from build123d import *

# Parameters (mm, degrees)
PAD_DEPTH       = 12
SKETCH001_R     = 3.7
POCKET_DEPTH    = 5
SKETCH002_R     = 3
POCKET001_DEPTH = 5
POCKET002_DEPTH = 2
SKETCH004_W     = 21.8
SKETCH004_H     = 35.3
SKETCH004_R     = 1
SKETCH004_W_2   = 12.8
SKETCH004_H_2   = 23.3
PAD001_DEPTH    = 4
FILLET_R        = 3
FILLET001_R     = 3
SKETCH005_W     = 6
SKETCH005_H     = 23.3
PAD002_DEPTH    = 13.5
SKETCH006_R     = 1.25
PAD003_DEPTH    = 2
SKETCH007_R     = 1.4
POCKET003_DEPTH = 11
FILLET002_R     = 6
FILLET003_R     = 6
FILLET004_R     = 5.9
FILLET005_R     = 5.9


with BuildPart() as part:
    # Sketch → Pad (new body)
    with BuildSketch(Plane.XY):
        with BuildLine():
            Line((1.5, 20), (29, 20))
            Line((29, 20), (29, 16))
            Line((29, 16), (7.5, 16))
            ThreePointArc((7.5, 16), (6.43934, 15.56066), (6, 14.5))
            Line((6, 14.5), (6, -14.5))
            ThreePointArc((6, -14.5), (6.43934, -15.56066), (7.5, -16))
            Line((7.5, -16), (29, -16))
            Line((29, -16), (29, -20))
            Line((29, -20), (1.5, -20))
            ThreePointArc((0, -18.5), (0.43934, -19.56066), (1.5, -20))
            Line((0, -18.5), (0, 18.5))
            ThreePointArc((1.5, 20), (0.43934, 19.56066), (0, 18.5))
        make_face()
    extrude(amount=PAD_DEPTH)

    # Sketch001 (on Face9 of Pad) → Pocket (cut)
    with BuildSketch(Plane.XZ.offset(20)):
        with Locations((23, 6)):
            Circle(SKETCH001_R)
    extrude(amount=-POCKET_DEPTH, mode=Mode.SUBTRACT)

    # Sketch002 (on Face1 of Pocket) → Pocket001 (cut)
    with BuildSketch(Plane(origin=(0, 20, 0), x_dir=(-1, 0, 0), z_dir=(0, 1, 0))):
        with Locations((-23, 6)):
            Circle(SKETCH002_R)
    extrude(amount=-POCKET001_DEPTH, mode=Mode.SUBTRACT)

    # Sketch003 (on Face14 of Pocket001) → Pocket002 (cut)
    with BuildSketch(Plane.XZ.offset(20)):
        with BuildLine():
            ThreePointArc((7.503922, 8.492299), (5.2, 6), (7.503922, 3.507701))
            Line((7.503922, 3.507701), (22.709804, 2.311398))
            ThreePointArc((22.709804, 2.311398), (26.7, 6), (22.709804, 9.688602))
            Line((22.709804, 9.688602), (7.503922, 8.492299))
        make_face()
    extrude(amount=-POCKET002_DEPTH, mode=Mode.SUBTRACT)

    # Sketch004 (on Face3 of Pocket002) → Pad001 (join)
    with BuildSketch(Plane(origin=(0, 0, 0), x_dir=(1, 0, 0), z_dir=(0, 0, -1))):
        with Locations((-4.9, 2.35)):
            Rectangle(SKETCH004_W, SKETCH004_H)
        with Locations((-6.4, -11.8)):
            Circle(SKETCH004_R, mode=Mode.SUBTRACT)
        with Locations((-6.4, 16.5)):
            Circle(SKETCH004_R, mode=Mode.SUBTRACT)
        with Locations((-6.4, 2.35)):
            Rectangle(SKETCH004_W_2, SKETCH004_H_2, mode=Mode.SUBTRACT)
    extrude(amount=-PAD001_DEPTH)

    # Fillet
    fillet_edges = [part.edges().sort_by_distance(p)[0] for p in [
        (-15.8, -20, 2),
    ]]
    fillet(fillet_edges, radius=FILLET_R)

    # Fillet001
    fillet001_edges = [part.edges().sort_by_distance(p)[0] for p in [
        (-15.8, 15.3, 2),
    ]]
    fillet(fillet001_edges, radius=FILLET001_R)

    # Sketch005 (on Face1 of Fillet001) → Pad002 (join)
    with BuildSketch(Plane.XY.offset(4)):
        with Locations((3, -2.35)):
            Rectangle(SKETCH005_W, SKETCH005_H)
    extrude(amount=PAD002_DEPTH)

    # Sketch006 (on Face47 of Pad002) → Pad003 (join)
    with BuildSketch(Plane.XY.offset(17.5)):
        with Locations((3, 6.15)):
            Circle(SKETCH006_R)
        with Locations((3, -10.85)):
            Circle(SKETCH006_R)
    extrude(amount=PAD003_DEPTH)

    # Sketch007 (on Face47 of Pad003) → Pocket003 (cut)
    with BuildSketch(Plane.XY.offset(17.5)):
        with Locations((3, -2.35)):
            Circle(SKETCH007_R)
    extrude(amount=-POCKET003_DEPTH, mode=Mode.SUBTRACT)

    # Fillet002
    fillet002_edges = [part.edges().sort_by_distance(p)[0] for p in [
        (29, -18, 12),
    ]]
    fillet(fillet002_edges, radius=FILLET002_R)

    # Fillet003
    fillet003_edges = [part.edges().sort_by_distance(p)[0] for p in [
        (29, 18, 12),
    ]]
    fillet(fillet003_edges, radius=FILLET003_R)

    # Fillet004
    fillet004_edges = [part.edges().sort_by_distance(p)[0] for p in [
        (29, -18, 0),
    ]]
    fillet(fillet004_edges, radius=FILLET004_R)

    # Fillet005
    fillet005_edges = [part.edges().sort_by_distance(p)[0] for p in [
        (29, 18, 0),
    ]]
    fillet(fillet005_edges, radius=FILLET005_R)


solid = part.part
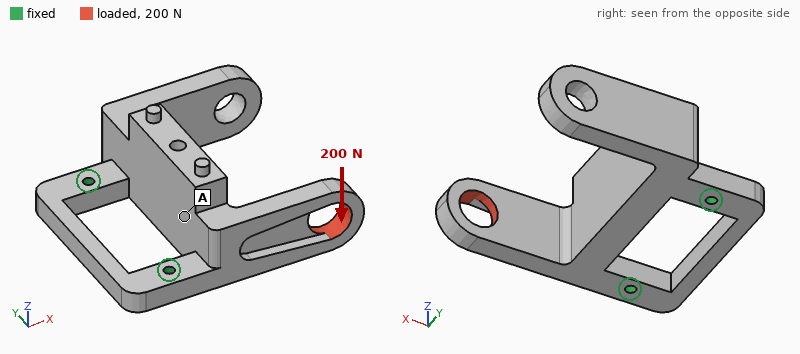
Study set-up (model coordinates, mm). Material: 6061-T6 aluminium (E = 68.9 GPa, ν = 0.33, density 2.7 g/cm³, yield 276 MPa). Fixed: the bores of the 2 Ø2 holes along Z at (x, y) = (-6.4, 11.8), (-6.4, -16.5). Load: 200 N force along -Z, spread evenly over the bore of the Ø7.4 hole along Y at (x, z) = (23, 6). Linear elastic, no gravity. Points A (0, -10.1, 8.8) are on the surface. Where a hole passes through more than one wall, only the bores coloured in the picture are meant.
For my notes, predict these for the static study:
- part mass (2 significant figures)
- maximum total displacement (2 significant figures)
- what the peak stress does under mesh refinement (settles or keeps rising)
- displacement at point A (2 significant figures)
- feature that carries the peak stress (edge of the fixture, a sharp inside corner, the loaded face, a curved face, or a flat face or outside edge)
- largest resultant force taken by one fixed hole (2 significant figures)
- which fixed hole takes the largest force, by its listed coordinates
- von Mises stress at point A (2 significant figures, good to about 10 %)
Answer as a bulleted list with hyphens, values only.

- 17 g
- 0.39 mm
- keeps rising
- 0.075 mm
- edge of the fixture
- 200 N
- (-6.4, -16.5)
- 25 MPa
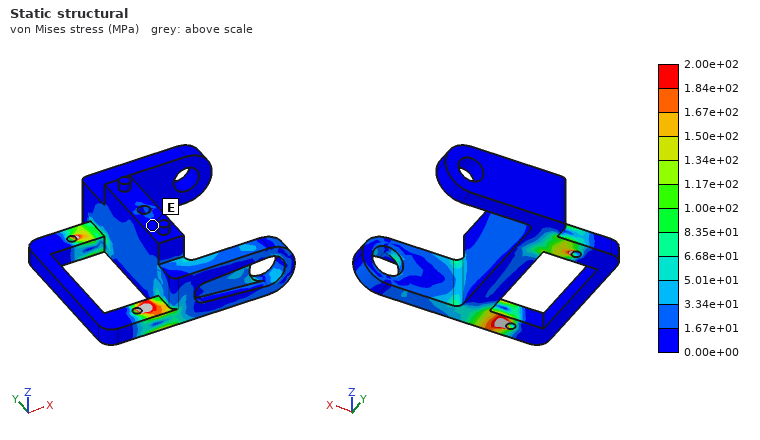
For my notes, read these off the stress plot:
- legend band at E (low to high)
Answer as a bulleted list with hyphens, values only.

- 0.00e+00 to 1.67e+01 MPa
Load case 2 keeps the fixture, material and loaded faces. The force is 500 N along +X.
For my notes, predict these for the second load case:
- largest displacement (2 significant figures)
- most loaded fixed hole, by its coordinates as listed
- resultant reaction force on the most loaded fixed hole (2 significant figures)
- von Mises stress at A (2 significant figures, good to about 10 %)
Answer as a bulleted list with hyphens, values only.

- 0.13 mm
- (-6.4, -16.5)
- 510 N
- 10 MPa
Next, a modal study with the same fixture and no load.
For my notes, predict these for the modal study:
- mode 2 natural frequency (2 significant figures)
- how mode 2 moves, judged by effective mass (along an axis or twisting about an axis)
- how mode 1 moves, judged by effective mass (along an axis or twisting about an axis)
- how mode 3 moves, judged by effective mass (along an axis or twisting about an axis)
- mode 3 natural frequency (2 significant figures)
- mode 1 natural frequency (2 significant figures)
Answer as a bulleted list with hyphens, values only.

- 4800 Hz
- along Y
- along Z
- along Y
- 5300 Hz
- 2200 Hz
